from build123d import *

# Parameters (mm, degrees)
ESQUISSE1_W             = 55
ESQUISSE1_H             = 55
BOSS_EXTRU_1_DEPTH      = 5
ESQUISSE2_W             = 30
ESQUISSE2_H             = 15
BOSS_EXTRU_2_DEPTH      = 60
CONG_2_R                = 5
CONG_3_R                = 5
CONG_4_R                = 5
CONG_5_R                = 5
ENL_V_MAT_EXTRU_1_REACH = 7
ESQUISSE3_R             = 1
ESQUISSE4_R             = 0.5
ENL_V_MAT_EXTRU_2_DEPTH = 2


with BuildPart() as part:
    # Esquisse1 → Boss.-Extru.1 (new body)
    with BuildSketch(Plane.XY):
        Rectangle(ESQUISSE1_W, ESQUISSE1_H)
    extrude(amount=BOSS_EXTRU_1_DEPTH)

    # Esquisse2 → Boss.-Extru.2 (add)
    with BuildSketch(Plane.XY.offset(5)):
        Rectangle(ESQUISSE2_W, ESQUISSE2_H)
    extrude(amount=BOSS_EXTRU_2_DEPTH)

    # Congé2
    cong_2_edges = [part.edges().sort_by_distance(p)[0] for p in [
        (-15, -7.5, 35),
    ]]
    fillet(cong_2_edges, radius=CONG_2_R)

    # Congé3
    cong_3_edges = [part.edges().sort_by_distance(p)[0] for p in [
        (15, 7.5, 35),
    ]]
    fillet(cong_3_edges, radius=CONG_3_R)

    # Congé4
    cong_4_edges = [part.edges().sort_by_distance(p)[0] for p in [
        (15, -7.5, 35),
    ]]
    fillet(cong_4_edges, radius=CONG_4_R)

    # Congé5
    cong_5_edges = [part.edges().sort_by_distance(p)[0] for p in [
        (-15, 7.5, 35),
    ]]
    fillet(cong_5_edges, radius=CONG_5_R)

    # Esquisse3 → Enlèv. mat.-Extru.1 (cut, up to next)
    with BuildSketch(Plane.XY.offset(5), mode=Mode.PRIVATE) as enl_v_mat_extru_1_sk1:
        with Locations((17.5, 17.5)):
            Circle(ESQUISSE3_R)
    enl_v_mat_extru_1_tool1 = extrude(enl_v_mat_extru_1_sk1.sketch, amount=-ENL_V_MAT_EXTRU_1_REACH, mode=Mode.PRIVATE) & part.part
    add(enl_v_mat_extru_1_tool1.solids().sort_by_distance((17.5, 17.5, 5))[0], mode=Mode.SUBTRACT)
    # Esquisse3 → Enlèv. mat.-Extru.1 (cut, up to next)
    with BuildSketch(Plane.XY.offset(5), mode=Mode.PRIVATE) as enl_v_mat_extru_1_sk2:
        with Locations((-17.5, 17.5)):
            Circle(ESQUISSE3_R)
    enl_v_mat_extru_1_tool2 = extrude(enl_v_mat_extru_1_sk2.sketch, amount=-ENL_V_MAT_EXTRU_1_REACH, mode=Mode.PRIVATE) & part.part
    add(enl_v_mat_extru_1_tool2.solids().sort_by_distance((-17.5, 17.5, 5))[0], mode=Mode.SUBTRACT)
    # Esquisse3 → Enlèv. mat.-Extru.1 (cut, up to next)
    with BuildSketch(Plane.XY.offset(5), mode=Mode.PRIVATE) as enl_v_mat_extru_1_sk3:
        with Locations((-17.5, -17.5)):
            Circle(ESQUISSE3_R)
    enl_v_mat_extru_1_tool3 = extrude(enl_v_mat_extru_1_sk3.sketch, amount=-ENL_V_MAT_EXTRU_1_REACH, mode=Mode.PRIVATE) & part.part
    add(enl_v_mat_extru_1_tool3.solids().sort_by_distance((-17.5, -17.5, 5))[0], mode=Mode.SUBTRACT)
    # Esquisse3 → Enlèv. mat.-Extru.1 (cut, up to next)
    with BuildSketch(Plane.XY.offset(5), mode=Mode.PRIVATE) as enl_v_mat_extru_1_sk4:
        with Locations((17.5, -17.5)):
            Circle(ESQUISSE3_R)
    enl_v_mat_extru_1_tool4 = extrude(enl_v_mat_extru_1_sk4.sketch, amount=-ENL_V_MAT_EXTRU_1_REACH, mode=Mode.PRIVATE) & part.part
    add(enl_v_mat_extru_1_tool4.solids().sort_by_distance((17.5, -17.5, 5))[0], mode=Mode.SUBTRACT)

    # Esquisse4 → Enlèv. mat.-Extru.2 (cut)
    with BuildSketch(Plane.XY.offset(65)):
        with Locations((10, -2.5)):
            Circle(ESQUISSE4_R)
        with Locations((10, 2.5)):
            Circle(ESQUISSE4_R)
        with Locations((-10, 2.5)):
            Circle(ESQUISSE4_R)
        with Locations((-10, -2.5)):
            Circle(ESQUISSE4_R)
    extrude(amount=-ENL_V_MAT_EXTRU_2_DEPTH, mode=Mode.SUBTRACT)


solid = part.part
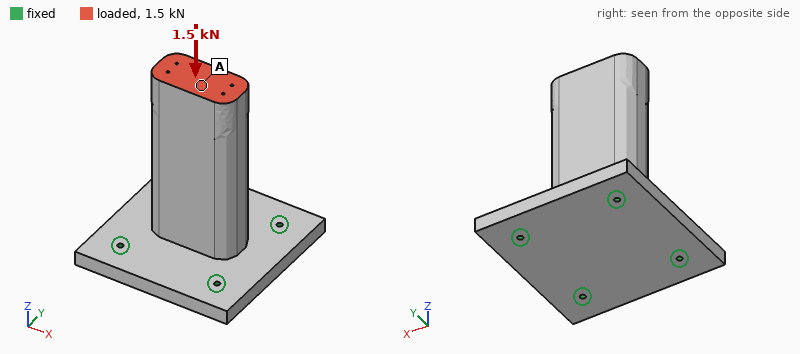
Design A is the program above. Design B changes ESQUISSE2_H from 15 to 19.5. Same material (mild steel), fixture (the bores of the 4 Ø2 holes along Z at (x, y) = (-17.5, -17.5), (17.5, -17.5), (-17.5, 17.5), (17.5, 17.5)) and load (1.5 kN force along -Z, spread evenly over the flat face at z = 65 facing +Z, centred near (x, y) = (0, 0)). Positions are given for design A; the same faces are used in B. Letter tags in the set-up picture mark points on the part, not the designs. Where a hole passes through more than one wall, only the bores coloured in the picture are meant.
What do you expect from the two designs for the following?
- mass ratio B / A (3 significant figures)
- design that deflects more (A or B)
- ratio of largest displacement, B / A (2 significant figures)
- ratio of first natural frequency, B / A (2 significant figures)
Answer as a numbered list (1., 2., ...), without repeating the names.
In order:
1. 1.20
2. A
3. 0.78
4. 1.1
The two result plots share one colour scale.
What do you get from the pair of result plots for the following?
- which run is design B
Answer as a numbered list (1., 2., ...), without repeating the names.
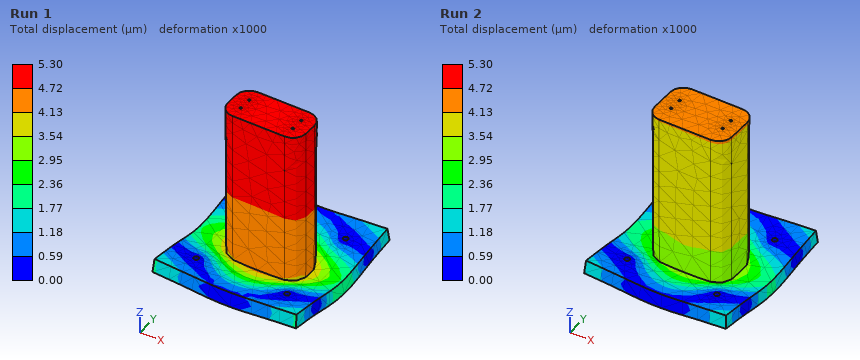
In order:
1. Run 2
